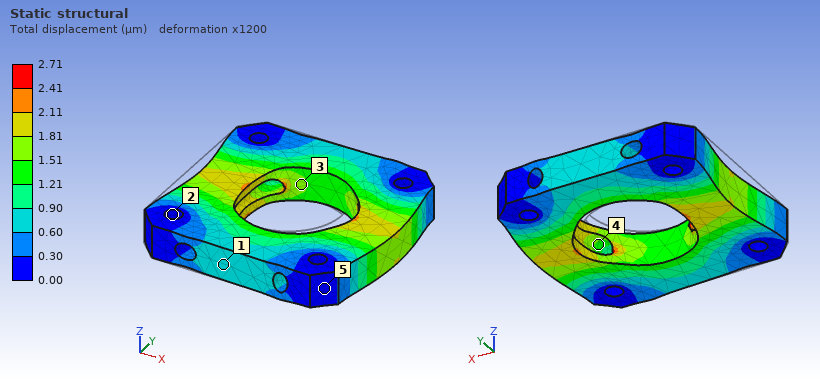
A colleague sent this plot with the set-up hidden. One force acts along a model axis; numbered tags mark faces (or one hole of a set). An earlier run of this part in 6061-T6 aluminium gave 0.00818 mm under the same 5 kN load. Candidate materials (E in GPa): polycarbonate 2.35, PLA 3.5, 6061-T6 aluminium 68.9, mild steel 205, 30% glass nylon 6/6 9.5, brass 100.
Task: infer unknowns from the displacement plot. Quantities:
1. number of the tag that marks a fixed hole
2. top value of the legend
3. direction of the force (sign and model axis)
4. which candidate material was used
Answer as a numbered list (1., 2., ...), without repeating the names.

1. 2
2. 2.71 µm
3. +X
4. mild steel
